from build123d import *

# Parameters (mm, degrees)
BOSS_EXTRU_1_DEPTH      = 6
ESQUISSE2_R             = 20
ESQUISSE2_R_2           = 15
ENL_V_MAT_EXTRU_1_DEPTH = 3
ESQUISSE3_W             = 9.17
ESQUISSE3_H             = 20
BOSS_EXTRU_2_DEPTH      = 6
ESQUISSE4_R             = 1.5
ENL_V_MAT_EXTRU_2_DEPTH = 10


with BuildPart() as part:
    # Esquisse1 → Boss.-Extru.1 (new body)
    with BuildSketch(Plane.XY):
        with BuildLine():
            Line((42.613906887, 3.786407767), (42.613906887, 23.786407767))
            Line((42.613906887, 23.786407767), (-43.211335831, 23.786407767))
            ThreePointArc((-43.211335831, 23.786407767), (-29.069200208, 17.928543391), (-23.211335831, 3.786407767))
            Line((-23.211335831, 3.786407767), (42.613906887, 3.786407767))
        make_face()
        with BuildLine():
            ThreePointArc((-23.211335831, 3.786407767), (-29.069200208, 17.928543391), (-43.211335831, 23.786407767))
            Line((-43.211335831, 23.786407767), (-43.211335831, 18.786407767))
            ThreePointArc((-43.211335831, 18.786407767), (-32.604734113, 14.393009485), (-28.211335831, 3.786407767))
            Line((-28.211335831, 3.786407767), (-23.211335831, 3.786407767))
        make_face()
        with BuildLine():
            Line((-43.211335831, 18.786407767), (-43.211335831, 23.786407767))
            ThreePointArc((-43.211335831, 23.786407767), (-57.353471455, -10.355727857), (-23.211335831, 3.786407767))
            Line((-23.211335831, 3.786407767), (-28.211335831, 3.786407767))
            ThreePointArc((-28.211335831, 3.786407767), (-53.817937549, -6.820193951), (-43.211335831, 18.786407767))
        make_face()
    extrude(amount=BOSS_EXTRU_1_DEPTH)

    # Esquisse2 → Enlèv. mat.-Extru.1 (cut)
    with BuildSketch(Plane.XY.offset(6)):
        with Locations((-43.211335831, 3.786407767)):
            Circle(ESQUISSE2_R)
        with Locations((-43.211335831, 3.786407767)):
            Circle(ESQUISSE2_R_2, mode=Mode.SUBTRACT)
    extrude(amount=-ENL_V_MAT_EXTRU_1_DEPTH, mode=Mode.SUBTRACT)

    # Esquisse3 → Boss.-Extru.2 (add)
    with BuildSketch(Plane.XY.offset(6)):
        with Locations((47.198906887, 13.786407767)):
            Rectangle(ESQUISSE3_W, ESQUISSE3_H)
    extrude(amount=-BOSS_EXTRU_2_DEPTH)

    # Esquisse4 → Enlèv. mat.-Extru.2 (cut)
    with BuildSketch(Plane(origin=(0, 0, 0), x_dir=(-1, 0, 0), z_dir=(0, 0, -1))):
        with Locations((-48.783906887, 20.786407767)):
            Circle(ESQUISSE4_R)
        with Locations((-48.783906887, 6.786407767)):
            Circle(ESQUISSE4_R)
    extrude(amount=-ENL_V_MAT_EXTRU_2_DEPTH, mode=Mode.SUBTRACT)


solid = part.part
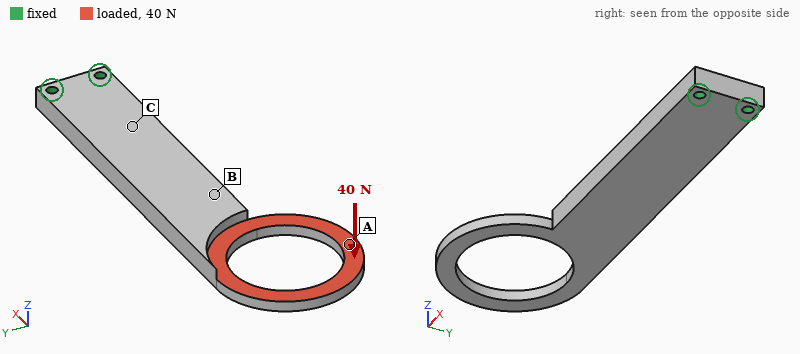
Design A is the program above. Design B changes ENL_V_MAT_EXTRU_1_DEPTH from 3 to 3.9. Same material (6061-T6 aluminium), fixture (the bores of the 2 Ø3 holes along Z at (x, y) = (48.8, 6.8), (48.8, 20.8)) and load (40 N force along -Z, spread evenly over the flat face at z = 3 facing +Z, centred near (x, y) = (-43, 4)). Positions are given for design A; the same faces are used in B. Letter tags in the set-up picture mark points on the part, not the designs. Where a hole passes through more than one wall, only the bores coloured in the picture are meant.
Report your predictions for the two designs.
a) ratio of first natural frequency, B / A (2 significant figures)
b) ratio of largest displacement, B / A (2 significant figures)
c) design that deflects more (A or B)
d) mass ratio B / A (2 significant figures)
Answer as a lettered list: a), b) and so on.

a) 1.1
b) 1.4
c) B
d) 0.96
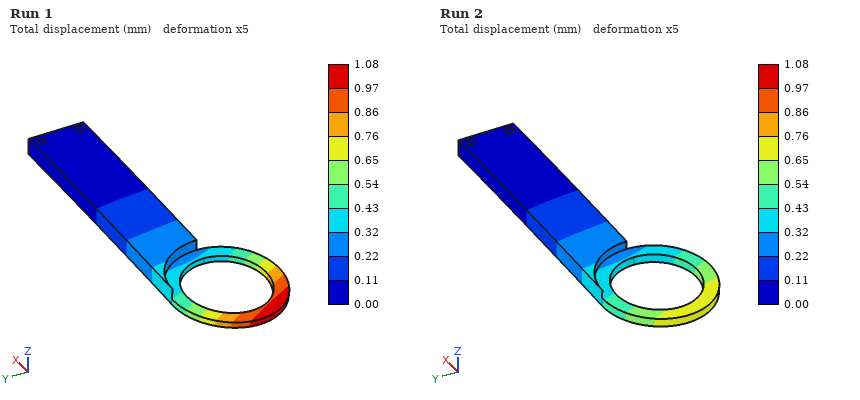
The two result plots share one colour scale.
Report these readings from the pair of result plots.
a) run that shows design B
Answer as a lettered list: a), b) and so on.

a) Run 1
